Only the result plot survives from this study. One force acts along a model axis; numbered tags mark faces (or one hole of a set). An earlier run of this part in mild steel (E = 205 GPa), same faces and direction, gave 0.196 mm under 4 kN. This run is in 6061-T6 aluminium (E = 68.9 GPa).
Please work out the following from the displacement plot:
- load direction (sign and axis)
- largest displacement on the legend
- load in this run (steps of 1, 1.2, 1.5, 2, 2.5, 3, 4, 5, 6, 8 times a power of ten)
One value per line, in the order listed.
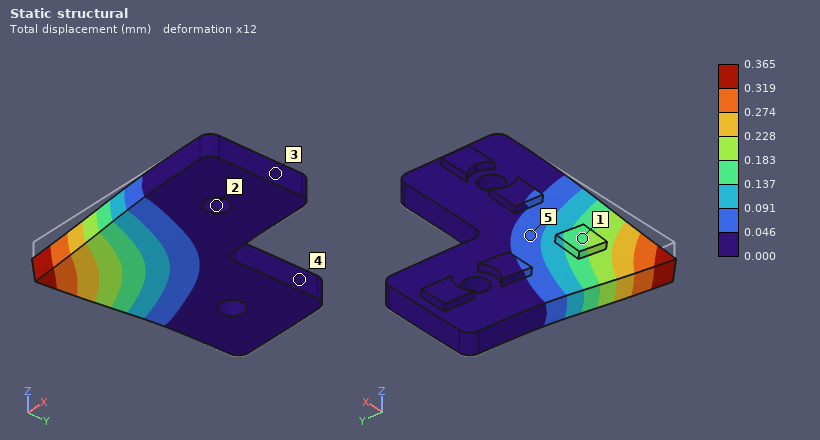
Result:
-Z
0.365 mm
2.5 kN
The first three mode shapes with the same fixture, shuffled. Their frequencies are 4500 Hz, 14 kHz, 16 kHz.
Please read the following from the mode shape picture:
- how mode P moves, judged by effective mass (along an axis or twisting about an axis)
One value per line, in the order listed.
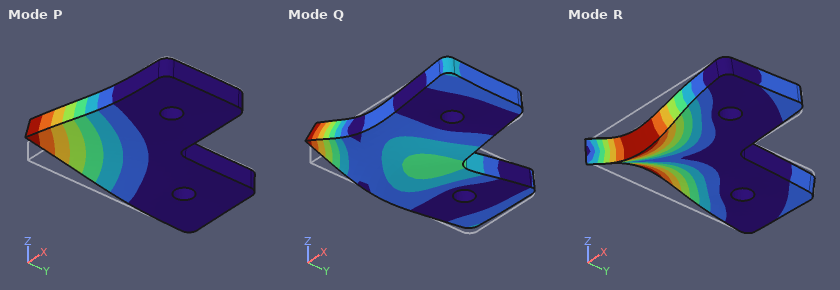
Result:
along Z
